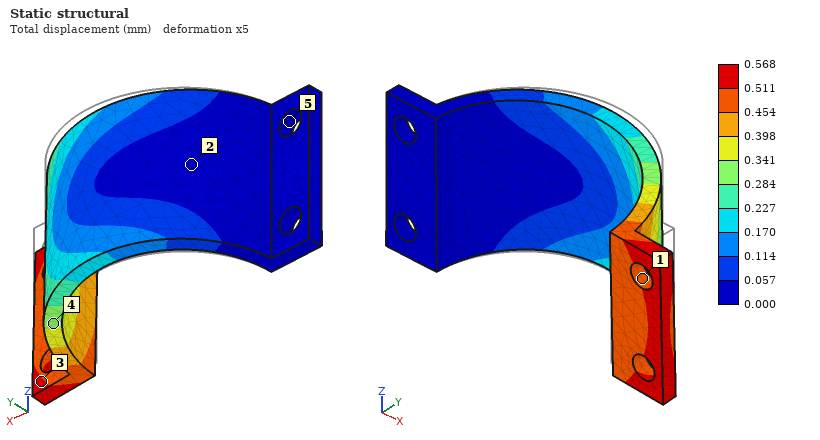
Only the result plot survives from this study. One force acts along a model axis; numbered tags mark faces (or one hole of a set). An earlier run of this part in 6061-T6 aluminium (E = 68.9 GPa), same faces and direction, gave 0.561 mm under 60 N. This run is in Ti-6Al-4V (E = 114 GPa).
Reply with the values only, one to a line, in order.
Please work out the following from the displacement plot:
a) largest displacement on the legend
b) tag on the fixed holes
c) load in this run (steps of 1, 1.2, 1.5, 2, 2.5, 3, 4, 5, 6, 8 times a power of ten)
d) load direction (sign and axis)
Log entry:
0.568 mm
5
100 N
-Z
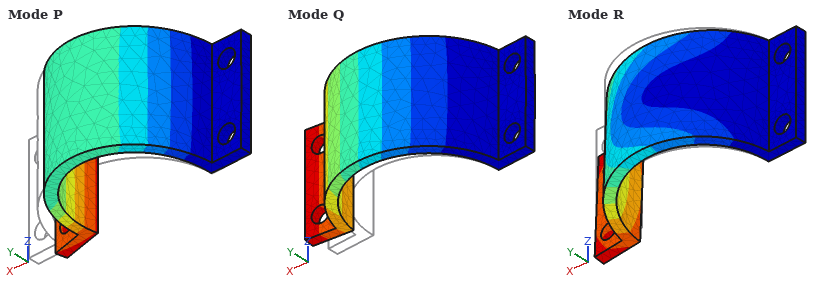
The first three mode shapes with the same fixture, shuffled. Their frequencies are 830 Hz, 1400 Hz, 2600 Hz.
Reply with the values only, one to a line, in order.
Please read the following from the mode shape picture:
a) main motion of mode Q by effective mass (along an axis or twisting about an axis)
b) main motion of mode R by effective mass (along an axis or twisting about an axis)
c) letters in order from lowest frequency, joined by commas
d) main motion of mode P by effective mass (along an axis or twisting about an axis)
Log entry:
along Y
along Z
Q, R, P
along X
